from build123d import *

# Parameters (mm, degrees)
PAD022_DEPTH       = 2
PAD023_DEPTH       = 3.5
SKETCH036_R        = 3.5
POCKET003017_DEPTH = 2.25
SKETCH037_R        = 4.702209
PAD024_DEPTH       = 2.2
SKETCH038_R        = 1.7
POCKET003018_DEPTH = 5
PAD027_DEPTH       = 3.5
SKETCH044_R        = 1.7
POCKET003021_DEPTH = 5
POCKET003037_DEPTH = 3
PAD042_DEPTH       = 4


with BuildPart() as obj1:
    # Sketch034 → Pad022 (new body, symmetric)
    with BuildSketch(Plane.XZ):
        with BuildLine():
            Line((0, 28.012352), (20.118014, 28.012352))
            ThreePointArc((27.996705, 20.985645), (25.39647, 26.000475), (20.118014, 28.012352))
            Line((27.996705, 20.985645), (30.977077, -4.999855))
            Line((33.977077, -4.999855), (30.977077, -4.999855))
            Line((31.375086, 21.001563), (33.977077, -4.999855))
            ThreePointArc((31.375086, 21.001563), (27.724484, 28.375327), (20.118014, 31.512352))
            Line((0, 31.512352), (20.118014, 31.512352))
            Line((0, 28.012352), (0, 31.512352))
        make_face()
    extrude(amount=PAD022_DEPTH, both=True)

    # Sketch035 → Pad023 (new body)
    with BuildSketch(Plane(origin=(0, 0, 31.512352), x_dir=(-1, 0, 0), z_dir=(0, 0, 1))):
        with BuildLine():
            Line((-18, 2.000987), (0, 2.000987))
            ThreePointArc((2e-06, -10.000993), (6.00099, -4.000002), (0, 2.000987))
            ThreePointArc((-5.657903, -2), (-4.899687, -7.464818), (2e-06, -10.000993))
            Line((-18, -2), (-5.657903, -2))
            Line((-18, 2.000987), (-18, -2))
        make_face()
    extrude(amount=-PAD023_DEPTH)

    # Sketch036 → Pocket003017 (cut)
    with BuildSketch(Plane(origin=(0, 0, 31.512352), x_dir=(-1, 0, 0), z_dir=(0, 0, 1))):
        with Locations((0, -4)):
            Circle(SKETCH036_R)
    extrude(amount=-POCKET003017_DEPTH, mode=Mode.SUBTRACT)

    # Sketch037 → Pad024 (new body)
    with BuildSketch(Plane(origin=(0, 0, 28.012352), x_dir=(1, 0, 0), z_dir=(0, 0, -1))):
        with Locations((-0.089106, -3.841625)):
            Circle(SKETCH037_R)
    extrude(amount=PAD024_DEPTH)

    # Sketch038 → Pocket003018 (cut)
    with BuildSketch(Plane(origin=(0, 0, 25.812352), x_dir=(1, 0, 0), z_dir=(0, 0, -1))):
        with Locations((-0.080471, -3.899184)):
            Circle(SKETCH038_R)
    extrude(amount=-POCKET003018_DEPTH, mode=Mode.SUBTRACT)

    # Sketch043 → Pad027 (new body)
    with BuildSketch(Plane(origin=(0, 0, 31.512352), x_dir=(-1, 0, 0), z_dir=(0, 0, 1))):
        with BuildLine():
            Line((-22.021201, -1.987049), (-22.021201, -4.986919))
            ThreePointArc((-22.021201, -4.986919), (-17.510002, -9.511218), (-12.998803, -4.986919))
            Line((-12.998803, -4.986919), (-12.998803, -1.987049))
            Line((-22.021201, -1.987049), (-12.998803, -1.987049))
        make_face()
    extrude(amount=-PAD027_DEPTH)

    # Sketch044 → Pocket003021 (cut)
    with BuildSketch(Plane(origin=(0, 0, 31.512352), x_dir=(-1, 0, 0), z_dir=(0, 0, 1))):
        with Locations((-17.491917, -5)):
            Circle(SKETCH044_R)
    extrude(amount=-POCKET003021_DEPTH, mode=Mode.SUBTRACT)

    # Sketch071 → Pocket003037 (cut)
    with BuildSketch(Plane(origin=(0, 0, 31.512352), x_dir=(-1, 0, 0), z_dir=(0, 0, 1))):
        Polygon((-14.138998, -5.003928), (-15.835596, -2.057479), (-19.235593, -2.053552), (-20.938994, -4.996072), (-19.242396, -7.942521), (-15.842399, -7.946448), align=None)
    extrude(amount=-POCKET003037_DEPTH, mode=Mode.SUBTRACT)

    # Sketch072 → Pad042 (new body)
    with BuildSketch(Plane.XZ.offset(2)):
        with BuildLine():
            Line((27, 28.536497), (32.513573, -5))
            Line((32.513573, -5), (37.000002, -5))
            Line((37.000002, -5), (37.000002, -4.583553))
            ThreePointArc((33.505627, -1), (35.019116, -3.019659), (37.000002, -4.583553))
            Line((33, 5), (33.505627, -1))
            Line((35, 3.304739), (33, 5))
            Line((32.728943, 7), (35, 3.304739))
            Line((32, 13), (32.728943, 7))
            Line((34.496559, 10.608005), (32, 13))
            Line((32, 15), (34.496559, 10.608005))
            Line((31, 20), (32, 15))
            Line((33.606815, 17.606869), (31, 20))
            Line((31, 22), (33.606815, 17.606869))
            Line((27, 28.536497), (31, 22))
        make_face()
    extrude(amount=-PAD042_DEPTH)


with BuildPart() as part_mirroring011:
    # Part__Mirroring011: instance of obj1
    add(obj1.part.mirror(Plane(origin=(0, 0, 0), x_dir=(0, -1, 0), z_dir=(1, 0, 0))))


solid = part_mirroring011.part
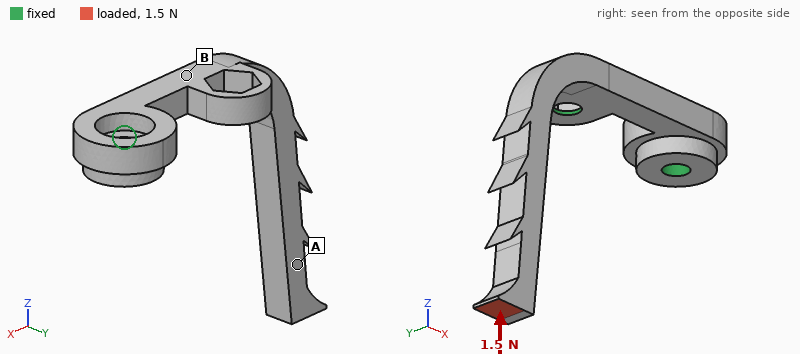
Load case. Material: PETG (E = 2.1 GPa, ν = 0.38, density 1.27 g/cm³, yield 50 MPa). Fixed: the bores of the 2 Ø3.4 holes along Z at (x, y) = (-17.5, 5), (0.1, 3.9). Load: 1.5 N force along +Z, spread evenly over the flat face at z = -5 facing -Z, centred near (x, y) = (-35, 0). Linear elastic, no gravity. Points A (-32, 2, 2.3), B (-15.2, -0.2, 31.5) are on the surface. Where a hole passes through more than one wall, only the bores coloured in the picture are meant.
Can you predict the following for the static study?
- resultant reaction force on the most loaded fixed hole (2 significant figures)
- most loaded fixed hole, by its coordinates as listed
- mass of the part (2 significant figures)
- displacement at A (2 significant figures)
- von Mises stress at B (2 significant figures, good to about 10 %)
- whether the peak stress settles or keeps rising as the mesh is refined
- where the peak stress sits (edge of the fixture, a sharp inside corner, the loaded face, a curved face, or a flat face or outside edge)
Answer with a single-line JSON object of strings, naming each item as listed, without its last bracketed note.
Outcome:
{"resultant reaction force on the most loaded fixed hole": "3.4 N", "most loaded fixed hole, by its coordinates as listed": "(-17.5, 5)", "mass of the part": "1.7 g", "displacement at A": "0.39 mm", "von Mises stress at B": "1.7 MPa", "whether the peak stress settles or keeps rising as the mesh is refined": "keeps rising", "where the peak stress sits": "edge of the fixture"}
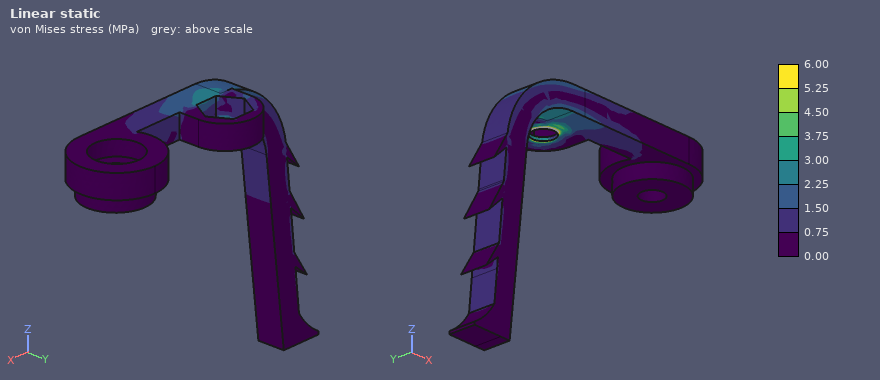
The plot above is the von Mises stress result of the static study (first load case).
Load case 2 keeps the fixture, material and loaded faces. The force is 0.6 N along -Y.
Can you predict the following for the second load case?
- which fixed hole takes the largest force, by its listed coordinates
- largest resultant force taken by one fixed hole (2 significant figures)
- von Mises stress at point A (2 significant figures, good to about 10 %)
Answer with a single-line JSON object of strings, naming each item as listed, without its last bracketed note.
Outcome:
{"which fixed hole takes the largest force, by its listed coordinates": "(-17.5, 5)", "largest resultant force taken by one fixed hole": "1.8 N", "von Mises stress at point A": "0.61 MPa"}
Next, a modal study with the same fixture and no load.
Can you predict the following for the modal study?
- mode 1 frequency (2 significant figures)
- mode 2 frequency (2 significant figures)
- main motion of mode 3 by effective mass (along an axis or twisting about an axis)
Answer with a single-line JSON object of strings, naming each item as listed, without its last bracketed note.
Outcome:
{"mode 1 frequency": "340 Hz", "mode 2 frequency": "370 Hz", "main motion of mode 3 by effective mass": "along Z"}
